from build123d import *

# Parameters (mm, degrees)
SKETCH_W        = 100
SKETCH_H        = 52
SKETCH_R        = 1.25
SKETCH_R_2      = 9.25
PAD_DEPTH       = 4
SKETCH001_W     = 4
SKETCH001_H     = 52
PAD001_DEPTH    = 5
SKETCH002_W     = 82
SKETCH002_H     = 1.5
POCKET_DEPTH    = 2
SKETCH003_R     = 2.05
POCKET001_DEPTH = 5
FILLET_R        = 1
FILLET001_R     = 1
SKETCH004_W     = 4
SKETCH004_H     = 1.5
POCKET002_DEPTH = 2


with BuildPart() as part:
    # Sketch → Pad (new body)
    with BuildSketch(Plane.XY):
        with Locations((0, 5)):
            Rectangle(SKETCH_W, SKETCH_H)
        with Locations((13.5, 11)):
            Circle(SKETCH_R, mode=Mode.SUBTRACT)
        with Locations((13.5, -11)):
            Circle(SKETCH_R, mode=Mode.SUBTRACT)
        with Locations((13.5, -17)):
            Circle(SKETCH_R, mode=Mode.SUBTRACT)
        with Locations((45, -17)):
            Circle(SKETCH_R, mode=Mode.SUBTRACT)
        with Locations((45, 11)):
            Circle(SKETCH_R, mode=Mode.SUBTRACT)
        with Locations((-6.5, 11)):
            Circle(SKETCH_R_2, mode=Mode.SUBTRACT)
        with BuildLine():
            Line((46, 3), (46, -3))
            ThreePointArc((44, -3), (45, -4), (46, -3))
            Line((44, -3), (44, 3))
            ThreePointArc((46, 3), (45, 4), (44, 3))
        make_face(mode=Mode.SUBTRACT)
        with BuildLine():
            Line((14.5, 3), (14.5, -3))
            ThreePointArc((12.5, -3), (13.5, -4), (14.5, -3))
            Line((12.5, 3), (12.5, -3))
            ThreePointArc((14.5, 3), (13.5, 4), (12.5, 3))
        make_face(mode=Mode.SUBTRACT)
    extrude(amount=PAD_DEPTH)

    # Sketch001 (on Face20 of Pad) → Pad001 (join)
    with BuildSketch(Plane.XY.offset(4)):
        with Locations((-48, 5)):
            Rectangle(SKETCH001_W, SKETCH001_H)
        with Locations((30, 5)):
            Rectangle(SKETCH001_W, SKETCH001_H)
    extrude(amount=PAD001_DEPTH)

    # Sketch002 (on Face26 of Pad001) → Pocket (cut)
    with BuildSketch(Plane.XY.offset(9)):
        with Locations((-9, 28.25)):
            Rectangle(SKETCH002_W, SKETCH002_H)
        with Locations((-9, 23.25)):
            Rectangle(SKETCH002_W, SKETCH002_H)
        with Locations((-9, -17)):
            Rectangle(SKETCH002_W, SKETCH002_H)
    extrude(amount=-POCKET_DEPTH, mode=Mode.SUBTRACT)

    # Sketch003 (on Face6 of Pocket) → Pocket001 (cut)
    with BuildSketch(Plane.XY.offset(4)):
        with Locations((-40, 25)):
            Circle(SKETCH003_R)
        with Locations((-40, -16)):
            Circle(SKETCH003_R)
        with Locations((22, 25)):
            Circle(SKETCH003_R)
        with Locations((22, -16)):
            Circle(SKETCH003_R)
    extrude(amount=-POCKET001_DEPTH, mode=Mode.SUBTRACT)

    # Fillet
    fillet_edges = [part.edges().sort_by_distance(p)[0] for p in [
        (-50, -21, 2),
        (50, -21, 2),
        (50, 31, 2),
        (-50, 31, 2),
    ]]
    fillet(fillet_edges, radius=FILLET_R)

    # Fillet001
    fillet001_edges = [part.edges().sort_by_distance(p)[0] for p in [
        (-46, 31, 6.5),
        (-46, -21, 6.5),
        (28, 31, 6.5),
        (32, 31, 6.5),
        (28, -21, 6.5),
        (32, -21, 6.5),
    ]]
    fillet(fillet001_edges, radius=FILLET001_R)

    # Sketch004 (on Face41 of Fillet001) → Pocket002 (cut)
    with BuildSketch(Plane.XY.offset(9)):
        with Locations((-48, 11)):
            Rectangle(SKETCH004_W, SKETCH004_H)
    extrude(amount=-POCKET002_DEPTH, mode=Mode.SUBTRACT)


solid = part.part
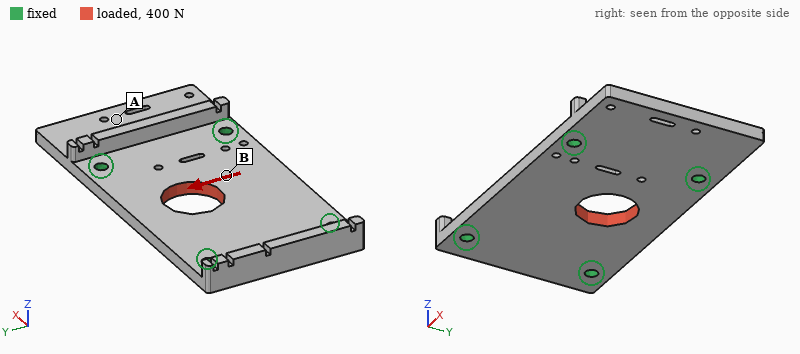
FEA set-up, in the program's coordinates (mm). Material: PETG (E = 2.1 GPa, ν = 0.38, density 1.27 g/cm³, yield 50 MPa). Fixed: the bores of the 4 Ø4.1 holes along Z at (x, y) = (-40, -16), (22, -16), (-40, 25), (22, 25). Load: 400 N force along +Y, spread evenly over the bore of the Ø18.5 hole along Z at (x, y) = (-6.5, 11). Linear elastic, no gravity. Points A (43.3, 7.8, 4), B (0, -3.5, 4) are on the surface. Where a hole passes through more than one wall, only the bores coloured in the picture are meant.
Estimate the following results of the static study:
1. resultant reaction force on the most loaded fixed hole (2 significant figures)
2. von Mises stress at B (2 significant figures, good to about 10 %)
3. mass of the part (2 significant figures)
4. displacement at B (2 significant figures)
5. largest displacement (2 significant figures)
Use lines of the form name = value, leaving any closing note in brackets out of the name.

resultant reaction force on the most loaded fixed hole = 130 N
von Mises stress at B = 1.6 MPa
mass of the part = 27 g
displacement at B = 38 µm
largest displacement = 65 µm
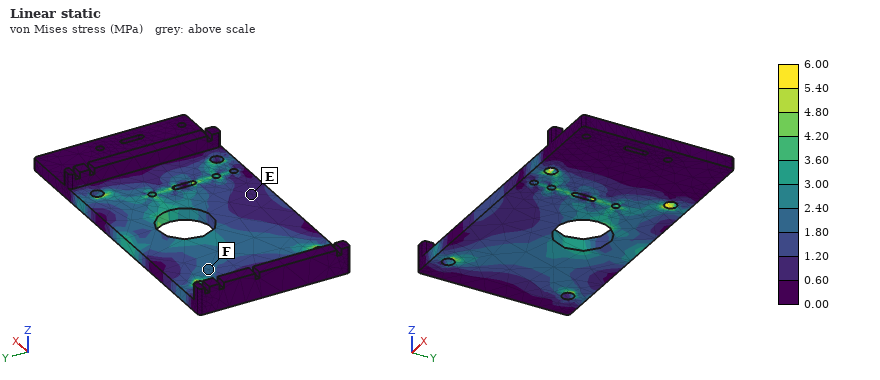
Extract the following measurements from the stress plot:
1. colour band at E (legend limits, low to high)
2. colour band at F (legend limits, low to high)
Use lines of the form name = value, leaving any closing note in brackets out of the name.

colour band at E = 0.60 to 1.20 MPa
colour band at F = 1.80 to 2.40 MPa
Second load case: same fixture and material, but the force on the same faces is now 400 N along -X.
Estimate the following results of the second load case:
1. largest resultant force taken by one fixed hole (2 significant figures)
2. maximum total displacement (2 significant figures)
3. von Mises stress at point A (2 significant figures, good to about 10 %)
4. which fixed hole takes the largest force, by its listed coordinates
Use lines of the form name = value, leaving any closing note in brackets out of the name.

largest resultant force taken by one fixed hole = 130 N
maximum total displacement = 25 µm
von Mises stress at point A = 0.32 MPa
which fixed hole takes the largest force, by its listed coordinates = (22, 25)
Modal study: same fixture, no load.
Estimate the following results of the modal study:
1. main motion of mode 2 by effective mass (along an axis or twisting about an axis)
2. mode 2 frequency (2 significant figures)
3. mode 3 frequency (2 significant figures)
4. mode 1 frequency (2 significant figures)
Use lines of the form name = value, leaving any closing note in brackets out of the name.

main motion of mode 2 by effective mass = along Z
mode 2 frequency = 1300 Hz
mode 3 frequency = 1700 Hz
mode 1 frequency = 970 Hz
